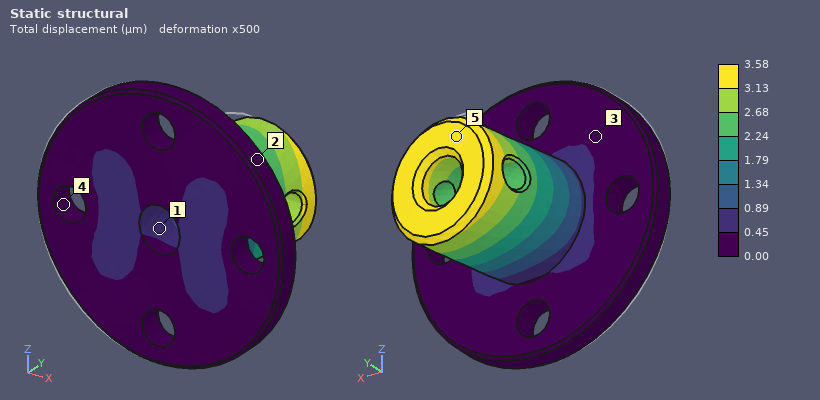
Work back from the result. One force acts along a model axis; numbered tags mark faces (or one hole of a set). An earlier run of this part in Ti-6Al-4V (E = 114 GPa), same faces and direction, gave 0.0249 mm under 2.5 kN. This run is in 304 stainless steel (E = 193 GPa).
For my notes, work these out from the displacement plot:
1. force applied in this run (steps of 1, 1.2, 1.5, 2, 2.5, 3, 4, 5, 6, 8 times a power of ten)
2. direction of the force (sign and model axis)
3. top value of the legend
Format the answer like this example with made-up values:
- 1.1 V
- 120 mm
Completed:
- 600 N
- +X
- 3.58 µm
